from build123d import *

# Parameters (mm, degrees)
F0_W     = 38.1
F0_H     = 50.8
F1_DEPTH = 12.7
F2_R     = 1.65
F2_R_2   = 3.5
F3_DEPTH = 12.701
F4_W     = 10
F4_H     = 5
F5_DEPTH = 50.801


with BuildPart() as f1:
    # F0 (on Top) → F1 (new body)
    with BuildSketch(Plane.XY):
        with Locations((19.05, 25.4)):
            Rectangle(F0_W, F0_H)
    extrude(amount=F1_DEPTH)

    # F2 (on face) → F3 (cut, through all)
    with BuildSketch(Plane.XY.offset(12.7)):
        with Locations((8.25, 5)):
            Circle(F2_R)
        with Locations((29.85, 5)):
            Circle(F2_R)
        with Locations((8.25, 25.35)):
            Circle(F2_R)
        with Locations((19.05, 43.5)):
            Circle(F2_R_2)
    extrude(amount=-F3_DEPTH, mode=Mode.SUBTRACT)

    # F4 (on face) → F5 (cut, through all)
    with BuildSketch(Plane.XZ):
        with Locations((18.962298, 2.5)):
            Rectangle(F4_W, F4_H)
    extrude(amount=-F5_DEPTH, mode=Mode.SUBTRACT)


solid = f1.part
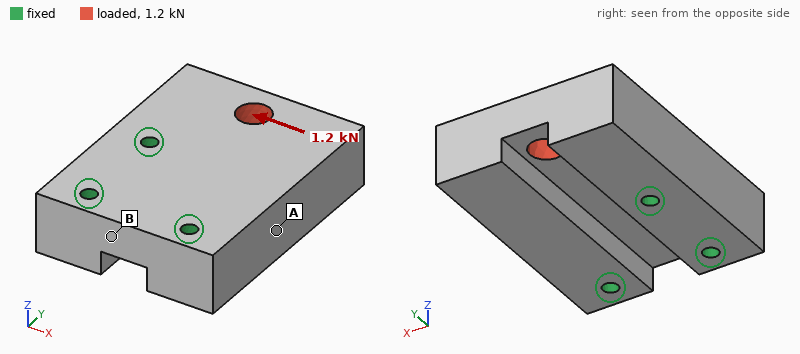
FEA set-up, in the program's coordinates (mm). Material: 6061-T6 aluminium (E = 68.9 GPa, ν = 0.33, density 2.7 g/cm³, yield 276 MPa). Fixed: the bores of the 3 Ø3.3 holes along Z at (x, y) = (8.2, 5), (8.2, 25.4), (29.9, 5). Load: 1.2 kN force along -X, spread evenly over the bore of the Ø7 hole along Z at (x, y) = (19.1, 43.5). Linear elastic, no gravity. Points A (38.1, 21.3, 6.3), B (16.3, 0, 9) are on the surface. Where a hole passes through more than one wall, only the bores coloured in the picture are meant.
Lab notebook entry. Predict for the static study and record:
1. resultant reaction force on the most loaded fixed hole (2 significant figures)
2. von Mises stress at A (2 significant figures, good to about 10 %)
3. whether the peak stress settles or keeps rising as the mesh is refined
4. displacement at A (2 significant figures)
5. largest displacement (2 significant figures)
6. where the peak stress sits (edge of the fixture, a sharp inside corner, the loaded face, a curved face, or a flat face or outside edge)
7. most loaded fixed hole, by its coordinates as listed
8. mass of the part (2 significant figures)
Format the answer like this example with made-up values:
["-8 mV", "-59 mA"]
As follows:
["1.4 kN", "6.5 MPa", "keeps rising", "2.6 µm", "8.5 µm", "edge of the fixture", "(8.2, 25.4)", "58 g"]
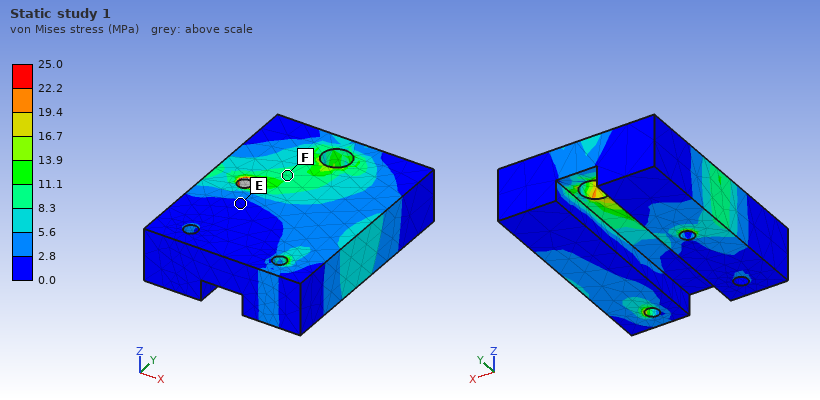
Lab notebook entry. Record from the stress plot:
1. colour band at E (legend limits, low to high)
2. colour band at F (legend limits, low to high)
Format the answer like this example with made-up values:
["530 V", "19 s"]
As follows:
["0.0 to 2.8 MPa", "8.3 to 11.1 MPa"]
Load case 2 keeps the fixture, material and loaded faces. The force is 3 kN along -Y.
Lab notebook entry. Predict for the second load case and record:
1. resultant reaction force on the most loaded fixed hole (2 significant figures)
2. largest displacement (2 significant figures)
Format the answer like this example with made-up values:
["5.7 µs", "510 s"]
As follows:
["1.4 kN", "13 µm"]
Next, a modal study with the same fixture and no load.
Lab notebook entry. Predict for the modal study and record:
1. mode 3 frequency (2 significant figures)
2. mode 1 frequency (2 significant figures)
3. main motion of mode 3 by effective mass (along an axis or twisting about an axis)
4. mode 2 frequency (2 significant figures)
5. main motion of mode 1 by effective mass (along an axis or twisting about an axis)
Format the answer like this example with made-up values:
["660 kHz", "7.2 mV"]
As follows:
["16 kHz", "7300 Hz", "along X", "14 kHz", "along Z"]
